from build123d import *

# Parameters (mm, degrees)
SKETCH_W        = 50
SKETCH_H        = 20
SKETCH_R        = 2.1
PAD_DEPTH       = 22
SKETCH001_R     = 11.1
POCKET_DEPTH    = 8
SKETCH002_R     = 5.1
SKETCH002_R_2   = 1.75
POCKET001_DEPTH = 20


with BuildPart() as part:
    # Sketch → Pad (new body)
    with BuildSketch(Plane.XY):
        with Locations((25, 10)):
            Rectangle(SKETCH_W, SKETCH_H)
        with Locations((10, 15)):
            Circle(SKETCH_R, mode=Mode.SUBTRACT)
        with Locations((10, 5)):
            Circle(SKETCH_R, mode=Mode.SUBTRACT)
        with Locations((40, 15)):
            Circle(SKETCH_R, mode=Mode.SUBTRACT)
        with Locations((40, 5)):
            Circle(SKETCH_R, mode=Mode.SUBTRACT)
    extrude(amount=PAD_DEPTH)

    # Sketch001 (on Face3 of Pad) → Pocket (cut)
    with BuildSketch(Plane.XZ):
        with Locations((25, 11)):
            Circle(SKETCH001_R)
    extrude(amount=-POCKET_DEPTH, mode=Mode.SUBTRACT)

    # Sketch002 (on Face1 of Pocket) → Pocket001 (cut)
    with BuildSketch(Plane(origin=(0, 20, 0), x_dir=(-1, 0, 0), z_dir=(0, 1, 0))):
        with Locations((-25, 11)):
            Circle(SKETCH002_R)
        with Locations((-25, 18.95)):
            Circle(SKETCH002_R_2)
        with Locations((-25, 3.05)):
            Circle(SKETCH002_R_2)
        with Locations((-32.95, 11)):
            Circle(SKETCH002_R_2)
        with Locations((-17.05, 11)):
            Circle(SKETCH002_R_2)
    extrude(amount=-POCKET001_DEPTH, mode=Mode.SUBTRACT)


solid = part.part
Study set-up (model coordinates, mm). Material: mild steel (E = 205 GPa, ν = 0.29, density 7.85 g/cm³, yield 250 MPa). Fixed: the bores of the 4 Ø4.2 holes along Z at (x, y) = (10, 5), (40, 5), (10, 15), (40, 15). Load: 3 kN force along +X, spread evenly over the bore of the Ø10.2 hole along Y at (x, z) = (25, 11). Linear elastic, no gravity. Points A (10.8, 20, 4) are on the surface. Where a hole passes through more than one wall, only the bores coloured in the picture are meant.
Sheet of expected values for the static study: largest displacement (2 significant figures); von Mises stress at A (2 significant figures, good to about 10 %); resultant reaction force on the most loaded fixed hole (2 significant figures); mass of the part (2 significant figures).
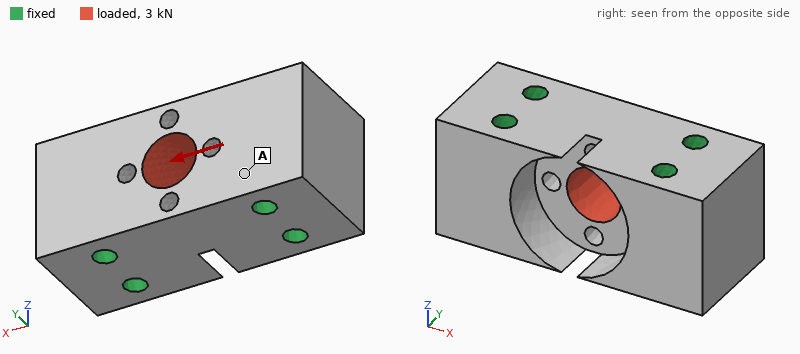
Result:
0.68 µm
3.4 MPa
1.2 kN
130 g
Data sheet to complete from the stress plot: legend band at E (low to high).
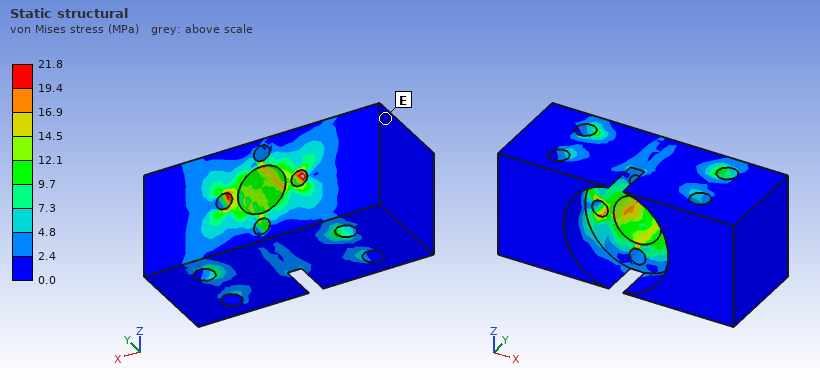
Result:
0.0 to 2.4 MPa
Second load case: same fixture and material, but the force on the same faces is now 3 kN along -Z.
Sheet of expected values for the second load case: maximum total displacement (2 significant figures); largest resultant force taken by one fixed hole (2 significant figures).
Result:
1.8 µm
1.1 kN
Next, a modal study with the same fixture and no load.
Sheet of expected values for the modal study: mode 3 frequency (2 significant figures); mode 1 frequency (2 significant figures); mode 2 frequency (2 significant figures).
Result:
60 kHz
55 kHz
55 kHz
